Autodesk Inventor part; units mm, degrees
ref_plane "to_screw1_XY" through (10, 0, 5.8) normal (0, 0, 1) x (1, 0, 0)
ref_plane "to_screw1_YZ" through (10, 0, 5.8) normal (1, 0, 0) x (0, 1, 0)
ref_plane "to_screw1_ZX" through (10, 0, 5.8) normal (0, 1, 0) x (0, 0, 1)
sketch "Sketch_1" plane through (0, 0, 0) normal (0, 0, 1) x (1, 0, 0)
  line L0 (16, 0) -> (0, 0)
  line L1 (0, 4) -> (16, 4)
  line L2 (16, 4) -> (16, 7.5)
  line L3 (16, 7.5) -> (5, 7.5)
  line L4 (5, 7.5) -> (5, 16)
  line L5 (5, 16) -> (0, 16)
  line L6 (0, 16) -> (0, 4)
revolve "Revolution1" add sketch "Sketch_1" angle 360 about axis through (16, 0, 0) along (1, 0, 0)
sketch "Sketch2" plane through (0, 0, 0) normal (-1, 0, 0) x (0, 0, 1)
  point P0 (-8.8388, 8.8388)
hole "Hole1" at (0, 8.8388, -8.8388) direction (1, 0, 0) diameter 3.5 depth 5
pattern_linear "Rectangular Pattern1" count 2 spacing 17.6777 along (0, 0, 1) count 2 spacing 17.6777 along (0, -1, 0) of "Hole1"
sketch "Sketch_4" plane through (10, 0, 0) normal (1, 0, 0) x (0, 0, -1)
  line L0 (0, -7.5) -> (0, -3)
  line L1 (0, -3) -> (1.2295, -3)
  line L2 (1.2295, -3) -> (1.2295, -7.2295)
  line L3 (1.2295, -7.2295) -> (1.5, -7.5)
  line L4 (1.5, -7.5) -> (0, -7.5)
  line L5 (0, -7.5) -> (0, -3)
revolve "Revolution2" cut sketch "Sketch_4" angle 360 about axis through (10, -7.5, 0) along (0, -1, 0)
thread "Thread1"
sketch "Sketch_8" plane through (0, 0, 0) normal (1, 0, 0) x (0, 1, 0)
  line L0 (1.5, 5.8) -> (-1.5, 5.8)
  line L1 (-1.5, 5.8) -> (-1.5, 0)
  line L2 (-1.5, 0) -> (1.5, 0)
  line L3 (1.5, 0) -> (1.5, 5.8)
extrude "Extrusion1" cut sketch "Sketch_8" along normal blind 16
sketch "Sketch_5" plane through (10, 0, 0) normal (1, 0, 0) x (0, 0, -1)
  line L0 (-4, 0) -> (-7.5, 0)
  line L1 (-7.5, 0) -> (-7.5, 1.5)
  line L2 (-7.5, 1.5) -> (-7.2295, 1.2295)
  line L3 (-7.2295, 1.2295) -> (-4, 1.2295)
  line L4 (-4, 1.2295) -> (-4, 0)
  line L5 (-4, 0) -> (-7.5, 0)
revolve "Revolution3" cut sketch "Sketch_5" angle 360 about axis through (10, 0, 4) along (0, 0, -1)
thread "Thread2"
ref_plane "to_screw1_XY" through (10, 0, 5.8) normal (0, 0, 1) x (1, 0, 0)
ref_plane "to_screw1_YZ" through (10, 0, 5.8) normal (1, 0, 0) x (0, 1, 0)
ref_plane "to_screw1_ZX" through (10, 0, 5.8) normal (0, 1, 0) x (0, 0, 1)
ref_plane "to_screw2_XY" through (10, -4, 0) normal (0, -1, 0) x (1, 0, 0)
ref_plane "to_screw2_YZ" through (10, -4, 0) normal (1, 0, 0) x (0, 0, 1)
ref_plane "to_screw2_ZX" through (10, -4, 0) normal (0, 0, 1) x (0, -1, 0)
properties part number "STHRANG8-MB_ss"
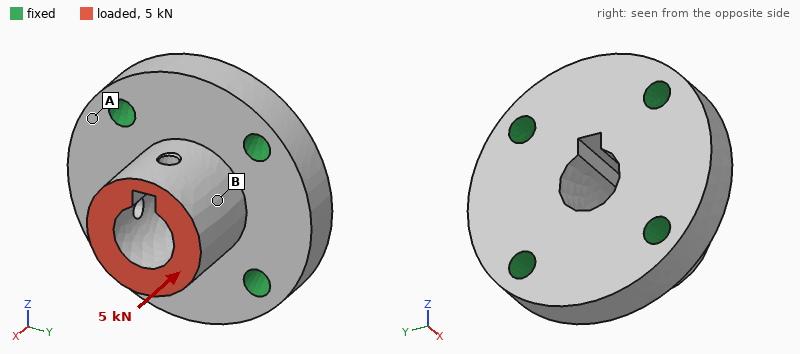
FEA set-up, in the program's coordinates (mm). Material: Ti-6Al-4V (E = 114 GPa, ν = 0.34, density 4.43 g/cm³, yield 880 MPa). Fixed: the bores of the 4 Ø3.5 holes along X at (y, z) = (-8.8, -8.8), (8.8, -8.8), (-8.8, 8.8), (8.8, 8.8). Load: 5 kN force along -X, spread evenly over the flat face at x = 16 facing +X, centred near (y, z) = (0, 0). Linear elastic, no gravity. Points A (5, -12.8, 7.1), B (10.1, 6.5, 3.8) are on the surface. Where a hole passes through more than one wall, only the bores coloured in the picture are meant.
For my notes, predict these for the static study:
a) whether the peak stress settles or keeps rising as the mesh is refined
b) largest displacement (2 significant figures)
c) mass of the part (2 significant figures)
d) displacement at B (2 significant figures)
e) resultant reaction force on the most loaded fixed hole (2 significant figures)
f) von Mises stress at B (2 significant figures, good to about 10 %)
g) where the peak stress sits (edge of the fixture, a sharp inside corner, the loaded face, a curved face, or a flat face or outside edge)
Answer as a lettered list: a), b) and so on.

a) keeps rising
b) 11 µm
c) 21 g
d) 8.1 µm
e) 1.3 kN
f) 38 MPa
g) edge of the fixture
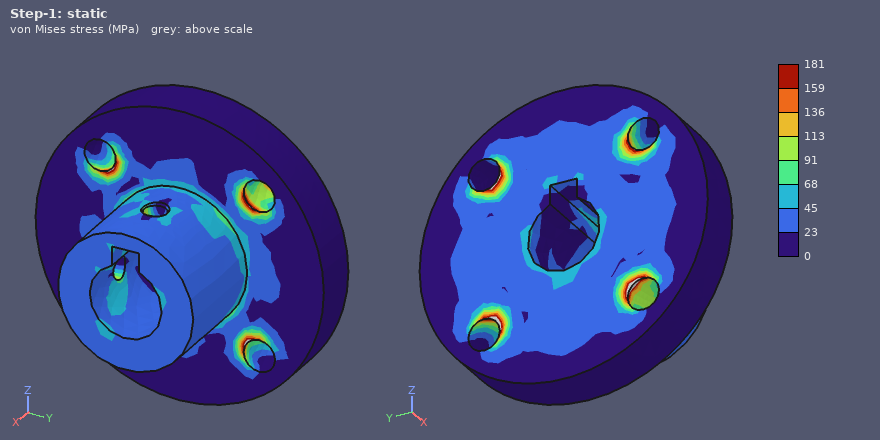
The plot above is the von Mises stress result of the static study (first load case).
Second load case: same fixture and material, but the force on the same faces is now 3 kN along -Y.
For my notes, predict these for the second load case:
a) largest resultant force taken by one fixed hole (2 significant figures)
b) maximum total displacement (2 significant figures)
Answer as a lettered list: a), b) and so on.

a) 1.6 kN
b) 40 µm
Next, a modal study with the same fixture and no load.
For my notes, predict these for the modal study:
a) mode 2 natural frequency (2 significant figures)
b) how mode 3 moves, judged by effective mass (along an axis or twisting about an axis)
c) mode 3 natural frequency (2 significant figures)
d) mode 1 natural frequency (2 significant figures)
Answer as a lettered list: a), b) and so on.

a) 32 kHz
b) along X
c) 43 kHz
d) 31 kHz
